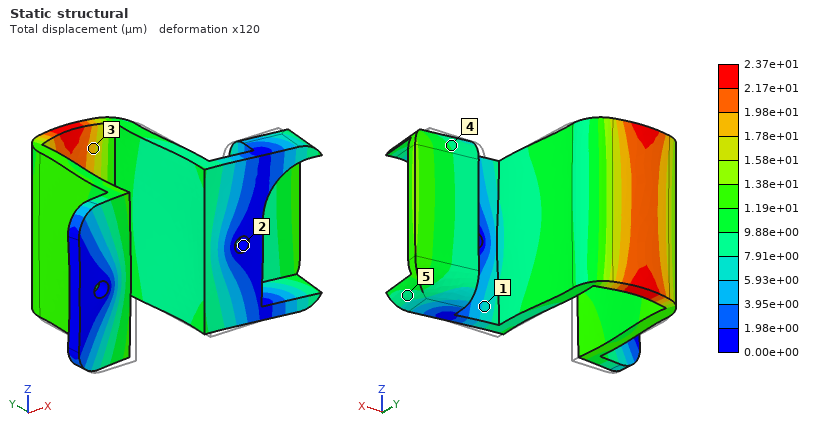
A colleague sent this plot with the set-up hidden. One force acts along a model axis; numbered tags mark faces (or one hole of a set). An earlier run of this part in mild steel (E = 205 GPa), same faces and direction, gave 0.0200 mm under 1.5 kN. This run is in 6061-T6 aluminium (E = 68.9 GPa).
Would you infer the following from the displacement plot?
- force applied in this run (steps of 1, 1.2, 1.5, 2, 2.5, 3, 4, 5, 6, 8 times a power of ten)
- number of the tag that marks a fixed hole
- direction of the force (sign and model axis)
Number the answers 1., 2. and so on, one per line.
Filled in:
1. 600 N
2. 2
3. +Y
